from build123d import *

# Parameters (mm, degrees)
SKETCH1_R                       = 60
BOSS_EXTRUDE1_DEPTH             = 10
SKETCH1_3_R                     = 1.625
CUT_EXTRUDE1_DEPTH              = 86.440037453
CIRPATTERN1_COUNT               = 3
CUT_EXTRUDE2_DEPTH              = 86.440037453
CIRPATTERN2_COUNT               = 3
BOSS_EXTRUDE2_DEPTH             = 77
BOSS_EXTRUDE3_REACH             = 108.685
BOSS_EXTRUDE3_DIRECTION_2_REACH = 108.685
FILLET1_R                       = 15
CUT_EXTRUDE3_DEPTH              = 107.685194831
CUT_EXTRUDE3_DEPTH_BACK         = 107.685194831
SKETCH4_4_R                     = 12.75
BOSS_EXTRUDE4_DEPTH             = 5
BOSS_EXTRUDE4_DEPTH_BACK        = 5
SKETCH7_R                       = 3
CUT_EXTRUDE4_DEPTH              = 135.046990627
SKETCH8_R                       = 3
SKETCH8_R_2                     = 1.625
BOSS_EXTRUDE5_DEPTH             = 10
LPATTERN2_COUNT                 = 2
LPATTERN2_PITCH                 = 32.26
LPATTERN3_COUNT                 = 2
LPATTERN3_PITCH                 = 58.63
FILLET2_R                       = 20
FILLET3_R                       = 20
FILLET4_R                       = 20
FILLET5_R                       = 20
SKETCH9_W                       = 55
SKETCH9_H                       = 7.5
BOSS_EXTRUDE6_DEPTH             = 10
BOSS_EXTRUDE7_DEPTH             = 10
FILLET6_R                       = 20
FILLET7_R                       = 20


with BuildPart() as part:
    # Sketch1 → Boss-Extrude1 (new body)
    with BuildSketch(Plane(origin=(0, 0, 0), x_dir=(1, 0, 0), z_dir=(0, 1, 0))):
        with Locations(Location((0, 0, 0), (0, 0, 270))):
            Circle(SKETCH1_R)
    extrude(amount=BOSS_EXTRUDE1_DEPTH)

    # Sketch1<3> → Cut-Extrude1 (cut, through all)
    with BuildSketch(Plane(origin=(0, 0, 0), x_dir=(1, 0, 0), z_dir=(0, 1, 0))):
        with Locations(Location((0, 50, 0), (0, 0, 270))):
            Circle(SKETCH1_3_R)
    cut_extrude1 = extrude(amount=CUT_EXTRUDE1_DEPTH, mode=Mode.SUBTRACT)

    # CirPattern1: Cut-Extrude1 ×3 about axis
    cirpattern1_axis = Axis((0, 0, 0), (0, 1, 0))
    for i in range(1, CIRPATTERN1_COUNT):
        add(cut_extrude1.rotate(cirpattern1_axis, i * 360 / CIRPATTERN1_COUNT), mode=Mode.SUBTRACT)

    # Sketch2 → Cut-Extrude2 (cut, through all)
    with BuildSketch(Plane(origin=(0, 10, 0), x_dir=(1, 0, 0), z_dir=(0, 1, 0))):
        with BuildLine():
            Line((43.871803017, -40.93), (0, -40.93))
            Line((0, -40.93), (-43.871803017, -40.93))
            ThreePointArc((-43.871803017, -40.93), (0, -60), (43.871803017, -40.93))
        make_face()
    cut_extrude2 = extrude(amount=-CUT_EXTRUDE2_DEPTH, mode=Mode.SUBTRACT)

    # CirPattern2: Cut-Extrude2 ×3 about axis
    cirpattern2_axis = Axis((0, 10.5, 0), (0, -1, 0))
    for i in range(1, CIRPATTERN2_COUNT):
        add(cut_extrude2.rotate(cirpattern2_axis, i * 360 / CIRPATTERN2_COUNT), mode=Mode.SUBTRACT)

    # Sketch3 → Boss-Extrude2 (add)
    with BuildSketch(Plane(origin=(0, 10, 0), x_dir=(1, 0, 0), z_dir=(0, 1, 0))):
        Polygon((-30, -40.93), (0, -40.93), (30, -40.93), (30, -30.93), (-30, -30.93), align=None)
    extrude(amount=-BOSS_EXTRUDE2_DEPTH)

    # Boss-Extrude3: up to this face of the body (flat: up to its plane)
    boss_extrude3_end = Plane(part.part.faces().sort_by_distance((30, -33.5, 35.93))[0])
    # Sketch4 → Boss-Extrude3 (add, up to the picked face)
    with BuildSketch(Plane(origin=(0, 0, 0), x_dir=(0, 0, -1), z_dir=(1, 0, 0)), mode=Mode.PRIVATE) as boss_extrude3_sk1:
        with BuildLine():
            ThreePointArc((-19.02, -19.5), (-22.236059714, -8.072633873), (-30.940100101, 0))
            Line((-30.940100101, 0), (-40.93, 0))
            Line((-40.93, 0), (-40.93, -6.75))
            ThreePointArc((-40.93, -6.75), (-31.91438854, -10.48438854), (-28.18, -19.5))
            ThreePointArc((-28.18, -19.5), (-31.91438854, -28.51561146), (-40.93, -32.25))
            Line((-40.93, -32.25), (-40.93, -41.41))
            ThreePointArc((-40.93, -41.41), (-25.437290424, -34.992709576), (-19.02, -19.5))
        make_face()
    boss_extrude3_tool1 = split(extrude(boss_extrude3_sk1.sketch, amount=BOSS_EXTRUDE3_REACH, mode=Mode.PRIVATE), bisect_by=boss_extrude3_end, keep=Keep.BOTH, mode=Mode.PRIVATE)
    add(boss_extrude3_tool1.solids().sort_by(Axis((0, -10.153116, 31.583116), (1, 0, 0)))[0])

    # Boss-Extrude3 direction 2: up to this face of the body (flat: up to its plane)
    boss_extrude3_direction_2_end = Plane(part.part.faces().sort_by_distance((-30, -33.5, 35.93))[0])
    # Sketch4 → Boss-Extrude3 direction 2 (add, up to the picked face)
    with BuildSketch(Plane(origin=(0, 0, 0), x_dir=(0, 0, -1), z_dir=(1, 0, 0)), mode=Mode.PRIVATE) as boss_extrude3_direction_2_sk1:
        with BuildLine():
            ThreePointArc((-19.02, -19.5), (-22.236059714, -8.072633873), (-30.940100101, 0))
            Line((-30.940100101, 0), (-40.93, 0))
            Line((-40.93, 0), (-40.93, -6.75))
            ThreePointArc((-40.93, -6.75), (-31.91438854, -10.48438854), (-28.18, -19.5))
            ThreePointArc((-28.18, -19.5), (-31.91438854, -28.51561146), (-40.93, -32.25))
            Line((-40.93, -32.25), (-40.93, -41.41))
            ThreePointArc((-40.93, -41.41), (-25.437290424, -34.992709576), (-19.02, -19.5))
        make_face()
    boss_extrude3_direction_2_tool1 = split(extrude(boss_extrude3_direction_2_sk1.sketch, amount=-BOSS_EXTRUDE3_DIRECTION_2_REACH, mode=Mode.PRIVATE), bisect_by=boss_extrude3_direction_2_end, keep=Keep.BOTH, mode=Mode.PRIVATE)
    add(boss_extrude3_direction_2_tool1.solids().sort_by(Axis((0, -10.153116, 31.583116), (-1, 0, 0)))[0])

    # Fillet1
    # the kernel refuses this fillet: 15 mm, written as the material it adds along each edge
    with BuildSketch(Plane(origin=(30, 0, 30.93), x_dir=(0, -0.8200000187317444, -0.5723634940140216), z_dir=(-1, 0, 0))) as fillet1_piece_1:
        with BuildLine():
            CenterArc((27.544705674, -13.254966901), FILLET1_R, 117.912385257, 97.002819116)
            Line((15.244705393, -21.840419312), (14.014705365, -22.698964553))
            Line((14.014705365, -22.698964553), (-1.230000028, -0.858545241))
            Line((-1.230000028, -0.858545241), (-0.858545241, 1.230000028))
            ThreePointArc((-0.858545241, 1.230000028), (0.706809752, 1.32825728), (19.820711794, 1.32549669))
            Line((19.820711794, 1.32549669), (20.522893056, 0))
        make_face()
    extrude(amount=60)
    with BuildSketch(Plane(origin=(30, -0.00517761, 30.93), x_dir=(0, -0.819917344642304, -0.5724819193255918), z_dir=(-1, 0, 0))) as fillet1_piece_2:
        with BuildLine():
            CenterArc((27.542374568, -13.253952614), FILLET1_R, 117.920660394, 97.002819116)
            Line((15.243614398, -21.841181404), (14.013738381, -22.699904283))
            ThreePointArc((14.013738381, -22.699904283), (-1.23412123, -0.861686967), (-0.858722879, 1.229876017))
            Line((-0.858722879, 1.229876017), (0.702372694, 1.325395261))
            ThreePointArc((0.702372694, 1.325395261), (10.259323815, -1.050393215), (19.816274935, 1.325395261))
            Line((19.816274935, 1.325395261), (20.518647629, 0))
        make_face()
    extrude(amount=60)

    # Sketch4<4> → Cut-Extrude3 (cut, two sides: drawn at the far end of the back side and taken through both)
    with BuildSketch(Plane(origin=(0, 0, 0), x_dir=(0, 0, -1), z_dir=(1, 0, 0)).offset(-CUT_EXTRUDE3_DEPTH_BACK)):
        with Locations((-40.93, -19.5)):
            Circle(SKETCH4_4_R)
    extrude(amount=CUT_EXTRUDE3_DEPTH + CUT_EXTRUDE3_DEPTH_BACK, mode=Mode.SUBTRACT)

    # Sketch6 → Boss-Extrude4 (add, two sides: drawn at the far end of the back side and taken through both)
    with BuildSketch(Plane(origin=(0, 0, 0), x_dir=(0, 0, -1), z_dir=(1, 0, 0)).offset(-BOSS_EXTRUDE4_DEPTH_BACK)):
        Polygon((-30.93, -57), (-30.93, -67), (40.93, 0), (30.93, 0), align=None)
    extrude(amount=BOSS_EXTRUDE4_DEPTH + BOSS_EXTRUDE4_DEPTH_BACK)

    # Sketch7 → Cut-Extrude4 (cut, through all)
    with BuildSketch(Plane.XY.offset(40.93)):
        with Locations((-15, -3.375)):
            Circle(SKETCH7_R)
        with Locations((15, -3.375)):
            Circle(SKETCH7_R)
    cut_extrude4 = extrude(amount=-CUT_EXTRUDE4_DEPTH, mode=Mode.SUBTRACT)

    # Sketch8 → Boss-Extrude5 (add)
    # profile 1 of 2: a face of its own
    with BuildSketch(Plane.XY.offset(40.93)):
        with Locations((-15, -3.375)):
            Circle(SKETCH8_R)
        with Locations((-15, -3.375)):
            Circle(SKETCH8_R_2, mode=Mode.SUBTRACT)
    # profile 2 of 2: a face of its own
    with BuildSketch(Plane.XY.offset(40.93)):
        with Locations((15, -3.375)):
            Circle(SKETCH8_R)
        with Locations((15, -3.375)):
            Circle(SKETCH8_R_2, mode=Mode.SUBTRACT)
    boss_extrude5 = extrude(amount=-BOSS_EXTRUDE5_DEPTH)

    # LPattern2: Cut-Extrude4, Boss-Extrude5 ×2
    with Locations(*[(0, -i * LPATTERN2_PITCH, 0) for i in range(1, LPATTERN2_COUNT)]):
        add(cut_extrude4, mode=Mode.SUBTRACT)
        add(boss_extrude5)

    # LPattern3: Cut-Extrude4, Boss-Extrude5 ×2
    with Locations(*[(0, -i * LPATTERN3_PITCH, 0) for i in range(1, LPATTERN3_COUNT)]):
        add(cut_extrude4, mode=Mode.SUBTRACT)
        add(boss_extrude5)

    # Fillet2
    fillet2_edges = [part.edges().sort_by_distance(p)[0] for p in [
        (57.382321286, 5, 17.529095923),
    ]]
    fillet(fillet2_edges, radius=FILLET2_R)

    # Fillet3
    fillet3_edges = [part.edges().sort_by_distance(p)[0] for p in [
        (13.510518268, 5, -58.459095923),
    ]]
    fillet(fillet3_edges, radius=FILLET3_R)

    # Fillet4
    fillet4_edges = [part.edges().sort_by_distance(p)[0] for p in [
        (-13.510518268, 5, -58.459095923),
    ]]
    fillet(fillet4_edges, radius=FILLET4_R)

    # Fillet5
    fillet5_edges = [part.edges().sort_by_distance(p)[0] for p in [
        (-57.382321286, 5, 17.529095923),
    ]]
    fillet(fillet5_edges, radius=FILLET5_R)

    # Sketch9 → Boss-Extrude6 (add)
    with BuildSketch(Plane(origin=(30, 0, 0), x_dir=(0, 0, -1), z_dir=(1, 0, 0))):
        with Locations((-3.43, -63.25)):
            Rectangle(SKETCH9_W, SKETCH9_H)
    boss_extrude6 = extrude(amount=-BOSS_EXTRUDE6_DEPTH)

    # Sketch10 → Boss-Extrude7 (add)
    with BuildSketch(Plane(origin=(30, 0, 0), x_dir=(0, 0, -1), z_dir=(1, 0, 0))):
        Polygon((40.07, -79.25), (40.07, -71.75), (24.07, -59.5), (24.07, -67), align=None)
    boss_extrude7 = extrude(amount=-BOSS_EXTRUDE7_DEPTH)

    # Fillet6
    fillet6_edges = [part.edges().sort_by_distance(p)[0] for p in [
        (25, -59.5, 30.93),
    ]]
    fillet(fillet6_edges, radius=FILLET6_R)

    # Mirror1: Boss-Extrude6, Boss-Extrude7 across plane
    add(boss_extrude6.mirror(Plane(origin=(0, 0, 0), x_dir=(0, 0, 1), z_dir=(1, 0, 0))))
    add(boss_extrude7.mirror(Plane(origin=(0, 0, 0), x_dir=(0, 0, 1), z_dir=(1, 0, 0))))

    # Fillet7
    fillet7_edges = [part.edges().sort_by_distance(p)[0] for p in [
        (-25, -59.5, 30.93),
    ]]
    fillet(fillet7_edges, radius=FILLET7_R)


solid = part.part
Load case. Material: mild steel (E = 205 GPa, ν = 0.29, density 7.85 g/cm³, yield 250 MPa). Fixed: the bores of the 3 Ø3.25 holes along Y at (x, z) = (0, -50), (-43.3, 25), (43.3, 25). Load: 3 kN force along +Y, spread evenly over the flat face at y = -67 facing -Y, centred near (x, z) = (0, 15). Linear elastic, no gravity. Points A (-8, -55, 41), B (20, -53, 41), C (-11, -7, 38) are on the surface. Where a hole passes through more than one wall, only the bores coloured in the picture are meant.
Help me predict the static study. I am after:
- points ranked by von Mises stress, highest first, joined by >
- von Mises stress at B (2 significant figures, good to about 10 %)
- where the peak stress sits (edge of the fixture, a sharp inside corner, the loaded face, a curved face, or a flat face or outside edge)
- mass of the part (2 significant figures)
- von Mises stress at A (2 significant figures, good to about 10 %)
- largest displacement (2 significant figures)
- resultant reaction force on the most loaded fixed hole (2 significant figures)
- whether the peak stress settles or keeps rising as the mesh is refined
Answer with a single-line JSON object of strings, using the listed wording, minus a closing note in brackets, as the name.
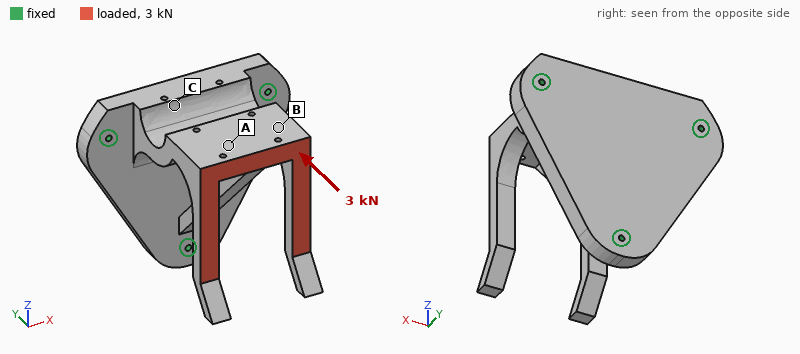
{"points ranked by von Mises stress, highest first, joined by >": "B > A > C", "von Mises stress at B": "39 MPa", "where the peak stress sits": "edge of the fixture", "mass of the part": "1.1 kg", "von Mises stress at A": "20 MPa", "largest displacement": "0.31 mm", "resultant reaction force on the most loaded fixed hole": "1.3 kN", "whether the peak stress settles or keeps rising as the mesh is refined": "keeps rising"}
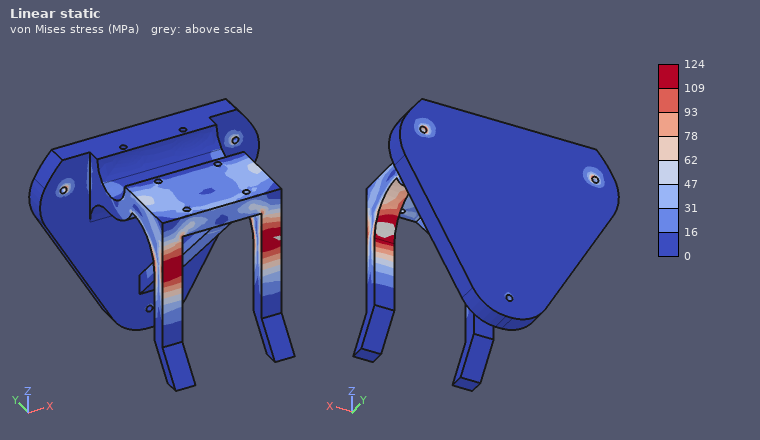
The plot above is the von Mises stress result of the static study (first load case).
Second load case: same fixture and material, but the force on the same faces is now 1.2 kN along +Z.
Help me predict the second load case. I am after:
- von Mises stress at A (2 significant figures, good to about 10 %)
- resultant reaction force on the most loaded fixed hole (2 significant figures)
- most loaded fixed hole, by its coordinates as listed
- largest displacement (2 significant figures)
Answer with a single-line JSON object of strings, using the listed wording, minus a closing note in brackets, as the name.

{"von Mises stress at A": "15 MPa", "resultant reaction force on the most loaded fixed hole": "1.4 kN", "most loaded fixed hole, by its coordinates as listed": "(0, -50)", "largest displacement": "80 µm"}
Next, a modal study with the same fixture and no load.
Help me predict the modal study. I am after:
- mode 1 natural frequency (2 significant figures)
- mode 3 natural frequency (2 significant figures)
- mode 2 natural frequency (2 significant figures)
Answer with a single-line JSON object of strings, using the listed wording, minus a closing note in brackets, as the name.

{"mode 1 natural frequency": "1200 Hz", "mode 3 natural frequency": "1400 Hz", "mode 2 natural frequency": "1300 Hz"}
